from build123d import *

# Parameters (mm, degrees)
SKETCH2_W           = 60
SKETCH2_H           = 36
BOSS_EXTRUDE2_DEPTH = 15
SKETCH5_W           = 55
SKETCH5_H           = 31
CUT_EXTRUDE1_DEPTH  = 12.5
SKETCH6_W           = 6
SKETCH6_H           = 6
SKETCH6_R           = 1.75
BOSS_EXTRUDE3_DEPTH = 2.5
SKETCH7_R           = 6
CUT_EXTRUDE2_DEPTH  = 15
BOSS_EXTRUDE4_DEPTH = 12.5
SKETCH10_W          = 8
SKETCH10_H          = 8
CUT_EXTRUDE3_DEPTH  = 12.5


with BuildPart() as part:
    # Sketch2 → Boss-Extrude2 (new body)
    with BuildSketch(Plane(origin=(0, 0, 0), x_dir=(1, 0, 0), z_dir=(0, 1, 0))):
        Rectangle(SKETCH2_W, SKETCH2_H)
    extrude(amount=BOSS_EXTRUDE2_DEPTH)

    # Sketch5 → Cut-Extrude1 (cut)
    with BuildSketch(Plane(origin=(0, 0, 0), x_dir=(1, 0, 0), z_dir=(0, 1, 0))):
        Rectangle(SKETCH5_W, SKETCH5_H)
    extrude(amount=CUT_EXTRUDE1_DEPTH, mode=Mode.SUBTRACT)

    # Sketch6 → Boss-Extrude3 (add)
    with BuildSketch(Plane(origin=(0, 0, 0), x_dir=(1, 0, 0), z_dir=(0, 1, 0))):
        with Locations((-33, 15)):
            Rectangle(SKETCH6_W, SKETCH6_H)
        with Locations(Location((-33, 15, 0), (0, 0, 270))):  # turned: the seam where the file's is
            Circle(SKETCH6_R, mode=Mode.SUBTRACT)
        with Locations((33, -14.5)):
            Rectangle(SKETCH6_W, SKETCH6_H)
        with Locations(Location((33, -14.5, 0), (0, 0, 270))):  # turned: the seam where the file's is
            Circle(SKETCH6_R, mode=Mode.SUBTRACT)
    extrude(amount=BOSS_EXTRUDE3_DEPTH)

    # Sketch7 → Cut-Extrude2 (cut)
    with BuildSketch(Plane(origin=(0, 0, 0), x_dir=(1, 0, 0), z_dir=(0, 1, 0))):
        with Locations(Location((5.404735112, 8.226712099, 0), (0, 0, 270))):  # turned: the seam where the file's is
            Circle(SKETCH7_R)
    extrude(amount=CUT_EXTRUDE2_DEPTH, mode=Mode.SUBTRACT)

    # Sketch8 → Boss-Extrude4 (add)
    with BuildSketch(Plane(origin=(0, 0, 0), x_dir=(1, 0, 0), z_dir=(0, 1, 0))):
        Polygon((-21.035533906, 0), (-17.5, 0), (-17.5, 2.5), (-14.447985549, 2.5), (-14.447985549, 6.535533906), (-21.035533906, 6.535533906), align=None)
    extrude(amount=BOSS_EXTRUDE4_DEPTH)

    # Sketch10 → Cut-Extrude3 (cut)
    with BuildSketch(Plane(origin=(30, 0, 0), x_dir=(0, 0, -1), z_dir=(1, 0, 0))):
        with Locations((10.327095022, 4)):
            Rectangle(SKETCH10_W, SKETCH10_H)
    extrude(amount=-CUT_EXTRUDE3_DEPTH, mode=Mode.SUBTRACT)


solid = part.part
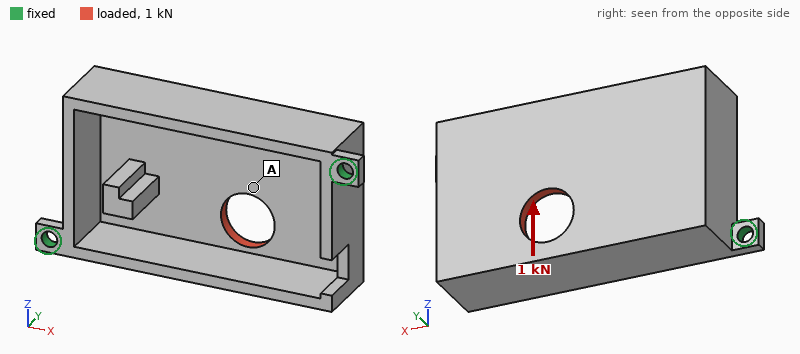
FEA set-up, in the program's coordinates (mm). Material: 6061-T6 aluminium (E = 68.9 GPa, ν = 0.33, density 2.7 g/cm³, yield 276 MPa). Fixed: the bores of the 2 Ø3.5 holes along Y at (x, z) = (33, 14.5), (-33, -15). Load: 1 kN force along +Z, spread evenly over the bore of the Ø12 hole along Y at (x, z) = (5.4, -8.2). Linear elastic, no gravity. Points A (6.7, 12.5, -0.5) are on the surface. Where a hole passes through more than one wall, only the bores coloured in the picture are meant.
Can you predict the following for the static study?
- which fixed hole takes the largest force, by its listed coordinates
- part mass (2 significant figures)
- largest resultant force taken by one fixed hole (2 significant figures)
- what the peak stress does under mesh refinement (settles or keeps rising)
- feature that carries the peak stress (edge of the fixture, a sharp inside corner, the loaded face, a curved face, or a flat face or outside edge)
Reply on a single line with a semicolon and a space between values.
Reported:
(33, 14.5); 30 g; 560 N; keeps rising; edge of the fixture
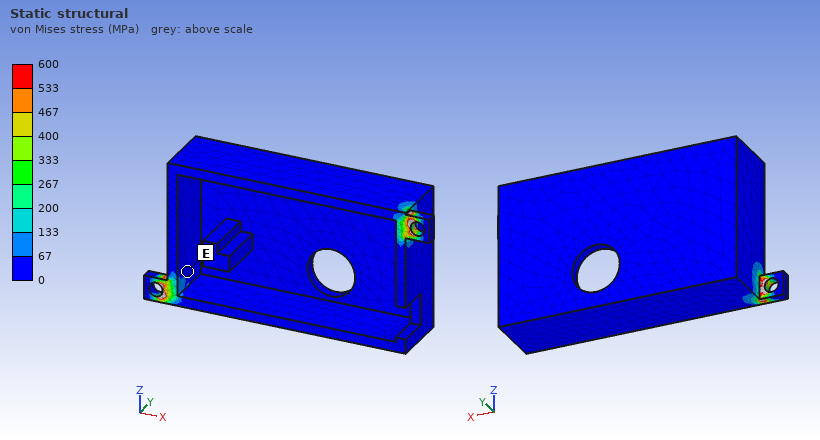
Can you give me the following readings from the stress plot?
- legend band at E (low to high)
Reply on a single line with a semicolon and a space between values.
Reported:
0 to 67 MPa
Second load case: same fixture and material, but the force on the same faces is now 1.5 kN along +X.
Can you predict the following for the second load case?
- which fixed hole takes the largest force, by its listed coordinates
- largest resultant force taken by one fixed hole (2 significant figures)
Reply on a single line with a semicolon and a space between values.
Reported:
(-33, -15); 980 N
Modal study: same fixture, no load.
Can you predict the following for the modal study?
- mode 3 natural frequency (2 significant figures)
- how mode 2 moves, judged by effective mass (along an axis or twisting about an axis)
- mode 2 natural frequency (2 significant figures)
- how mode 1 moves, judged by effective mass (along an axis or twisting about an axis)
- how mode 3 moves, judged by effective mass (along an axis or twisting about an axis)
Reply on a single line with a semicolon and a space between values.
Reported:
5700 Hz; along Y; 4900 Hz; along Z; along Z
